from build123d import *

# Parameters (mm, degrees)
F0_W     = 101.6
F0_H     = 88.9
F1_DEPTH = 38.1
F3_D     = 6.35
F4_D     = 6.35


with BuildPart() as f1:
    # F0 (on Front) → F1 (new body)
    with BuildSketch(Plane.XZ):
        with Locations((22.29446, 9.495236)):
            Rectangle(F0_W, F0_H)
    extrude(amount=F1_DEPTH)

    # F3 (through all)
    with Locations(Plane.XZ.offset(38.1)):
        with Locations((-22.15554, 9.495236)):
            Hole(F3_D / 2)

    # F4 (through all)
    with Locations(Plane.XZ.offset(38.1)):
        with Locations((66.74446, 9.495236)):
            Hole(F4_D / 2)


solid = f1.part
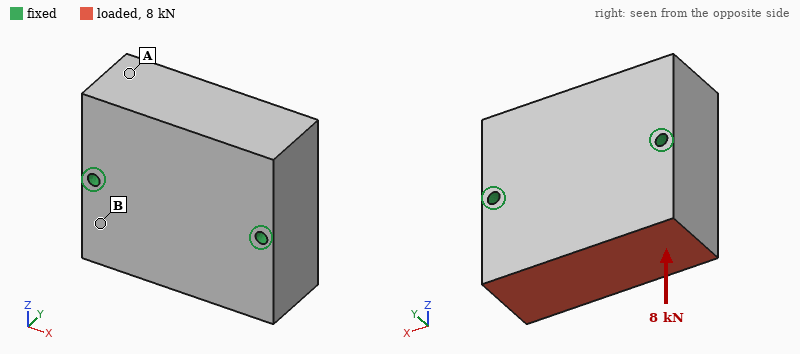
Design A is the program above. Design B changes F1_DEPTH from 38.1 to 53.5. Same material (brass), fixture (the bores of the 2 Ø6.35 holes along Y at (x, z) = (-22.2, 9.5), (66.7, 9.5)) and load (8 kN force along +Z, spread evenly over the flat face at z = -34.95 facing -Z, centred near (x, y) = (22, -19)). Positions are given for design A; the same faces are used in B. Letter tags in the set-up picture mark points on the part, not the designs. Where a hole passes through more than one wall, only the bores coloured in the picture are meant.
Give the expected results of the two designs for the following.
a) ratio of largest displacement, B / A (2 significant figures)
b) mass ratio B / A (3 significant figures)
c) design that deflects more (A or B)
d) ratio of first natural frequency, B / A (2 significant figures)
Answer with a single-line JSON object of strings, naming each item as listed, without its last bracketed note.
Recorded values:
{"ratio of largest displacement, B / A": "0.72", "mass ratio B / A": "1.40", "design that deflects more": "A", "ratio of first natural frequency, B / A": "1.2"}
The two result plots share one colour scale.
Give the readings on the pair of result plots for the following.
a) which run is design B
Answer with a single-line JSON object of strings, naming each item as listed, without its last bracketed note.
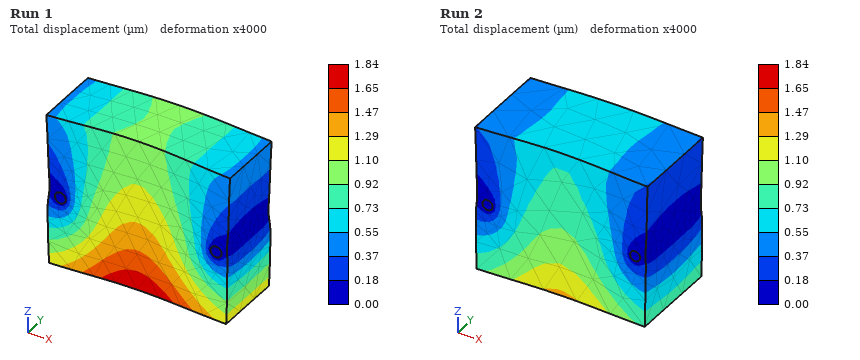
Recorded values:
{"which run is design B": "Run 2"}
